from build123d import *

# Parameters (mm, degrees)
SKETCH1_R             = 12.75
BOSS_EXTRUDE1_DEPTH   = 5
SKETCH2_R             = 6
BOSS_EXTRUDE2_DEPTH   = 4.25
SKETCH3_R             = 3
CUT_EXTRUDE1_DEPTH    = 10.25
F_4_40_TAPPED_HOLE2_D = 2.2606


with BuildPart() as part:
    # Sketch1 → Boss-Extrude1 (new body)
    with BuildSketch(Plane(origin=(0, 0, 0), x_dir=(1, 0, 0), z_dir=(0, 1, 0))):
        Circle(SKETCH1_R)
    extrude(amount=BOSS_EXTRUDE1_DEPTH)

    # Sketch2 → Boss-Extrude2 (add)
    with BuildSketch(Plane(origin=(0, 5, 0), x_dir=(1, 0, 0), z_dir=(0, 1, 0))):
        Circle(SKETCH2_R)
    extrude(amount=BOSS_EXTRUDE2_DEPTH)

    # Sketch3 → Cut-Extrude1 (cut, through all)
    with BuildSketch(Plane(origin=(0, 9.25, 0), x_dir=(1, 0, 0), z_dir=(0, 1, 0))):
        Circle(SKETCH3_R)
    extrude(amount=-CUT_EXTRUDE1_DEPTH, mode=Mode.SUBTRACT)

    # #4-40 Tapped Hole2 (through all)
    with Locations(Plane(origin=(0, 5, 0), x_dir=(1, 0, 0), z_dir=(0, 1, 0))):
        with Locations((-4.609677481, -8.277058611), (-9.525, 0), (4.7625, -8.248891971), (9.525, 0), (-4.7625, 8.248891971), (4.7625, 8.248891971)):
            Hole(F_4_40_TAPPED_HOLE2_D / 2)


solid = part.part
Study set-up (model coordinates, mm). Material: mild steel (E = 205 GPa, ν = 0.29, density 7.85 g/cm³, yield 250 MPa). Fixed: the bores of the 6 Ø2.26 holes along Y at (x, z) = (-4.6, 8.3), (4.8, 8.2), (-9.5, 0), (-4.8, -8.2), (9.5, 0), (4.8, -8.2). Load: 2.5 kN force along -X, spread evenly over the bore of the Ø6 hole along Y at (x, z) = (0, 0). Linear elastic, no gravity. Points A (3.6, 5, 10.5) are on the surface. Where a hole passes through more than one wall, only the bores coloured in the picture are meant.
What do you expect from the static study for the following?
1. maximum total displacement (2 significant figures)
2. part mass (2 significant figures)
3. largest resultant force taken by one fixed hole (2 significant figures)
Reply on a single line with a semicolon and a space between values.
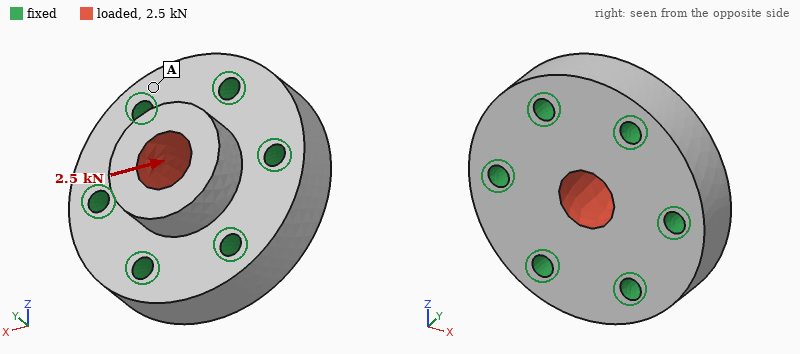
1.9 µm; 21 g; 650 N
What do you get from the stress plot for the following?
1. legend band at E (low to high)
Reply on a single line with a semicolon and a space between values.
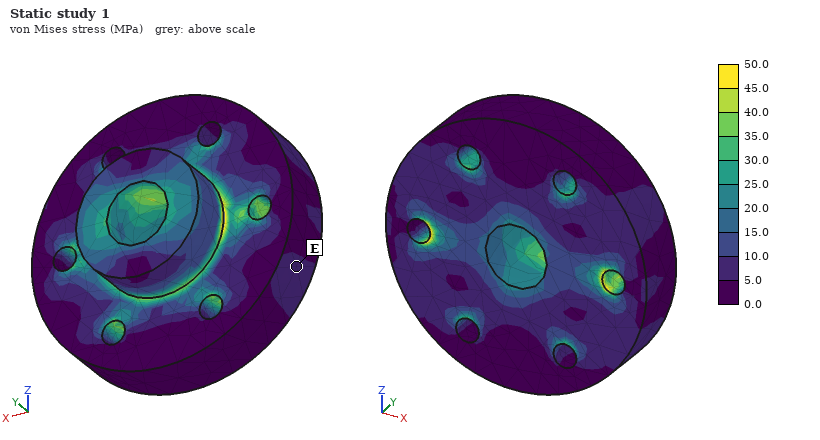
5.0 to 10.0 MPa
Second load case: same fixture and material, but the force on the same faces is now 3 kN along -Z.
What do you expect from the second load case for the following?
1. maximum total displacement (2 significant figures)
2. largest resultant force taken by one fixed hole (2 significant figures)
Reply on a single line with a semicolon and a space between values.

2.2 µm; 700 N
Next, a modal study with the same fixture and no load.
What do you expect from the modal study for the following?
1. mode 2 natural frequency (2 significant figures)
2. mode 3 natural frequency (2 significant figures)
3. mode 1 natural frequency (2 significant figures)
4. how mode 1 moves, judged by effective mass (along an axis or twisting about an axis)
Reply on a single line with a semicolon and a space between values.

90 kHz; 90 kHz; 84 kHz; along Y
